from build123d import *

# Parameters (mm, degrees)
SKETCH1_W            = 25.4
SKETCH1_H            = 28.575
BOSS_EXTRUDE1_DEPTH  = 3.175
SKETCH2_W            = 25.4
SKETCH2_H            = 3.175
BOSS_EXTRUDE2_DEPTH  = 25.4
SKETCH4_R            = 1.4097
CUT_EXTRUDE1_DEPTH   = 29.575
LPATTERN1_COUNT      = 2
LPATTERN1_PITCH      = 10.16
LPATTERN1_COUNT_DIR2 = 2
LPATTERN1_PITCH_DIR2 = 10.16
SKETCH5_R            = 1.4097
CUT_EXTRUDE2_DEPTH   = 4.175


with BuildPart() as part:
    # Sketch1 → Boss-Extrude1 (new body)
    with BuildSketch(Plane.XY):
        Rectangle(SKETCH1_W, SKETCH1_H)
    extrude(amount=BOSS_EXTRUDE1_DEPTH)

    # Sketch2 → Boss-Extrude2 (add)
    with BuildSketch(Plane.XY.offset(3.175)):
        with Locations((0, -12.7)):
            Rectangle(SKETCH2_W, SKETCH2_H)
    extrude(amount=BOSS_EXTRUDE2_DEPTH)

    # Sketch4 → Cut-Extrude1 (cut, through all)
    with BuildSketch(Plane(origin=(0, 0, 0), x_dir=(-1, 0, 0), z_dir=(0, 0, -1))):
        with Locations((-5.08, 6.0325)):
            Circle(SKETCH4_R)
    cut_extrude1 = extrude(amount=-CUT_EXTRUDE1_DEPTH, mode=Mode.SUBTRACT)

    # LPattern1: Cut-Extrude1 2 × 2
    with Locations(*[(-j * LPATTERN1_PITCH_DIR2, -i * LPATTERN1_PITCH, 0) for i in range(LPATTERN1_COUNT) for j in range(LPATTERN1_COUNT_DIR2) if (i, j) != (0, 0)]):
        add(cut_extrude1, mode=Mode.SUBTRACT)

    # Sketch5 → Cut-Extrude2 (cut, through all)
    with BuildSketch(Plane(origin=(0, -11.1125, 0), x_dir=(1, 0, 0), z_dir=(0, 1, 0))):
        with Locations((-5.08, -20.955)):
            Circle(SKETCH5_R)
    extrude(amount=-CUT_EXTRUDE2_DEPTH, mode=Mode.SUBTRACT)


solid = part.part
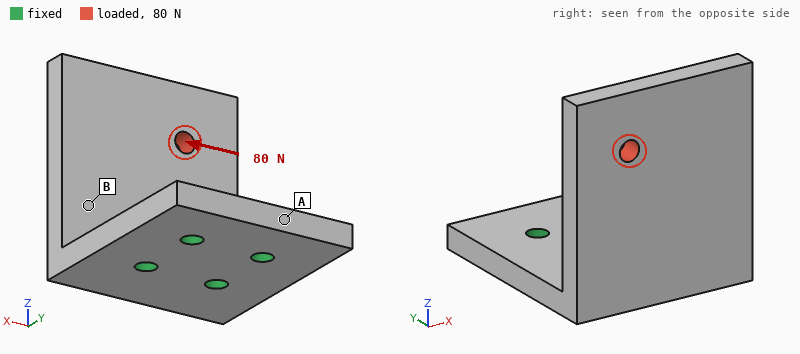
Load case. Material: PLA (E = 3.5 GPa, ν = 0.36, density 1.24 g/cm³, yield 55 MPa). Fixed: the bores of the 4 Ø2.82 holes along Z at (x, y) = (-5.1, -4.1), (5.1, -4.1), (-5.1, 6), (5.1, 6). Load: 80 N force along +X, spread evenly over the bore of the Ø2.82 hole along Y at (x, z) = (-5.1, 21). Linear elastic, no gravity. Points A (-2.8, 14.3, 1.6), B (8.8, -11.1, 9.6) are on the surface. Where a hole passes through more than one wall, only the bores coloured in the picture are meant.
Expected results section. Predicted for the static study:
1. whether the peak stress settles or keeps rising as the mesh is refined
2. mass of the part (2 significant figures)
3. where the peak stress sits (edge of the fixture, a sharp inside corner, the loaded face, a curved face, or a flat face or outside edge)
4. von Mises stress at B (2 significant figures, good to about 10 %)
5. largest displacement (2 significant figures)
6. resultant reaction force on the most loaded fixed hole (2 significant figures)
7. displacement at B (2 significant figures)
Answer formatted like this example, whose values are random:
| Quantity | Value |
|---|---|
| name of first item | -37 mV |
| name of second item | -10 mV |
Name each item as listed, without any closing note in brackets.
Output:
| Quantity | Value |
|---|---|
| whether the peak stress settles or keeps rising as the mesh is refined | keeps rising |
| mass of the part | 5.3 g |
| where the peak stress sits | edge of the fixture |
| von Mises stress at B | 6.7 MPa |
| largest displacement | 0.48 mm |
| resultant reaction force on the most loaded fixed hole | 130 N |
| displacement at B | 0.19 mm |
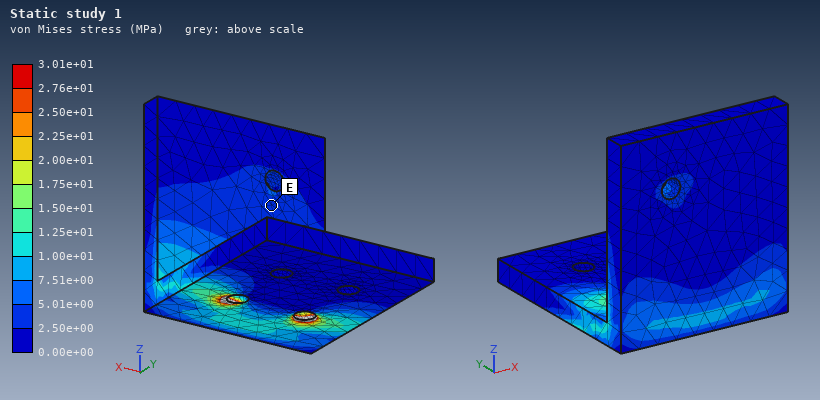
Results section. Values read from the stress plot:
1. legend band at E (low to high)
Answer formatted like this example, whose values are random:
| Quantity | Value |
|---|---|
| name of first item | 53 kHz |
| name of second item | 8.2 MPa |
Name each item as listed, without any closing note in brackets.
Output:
| Quantity | Value |
|---|---|
| legend band at E | 2.50e+00 to 5.01e+00 MPa |
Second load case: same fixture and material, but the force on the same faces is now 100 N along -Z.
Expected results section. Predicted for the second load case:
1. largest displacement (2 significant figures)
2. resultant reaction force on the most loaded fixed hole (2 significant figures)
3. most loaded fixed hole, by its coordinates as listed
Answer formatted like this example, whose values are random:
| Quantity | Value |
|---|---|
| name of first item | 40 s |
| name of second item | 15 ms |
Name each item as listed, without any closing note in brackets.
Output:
| Quantity | Value |
|---|---|
| largest displacement | 0.49 mm |
| resultant reaction force on the most loaded fixed hole | 98 N |
| most loaded fixed hole, by its coordinates as listed | (-5.1, -4.1) |
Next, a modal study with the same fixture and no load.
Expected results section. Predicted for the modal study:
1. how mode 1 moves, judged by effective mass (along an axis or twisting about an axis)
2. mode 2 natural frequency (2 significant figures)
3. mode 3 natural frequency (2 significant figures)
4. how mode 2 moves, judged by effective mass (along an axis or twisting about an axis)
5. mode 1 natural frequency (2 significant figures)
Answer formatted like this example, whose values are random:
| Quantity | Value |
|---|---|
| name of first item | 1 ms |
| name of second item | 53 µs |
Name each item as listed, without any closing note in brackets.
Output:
| Quantity | Value |
|---|---|
| how mode 1 moves, judged by effective mass | along Y |
| mode 2 natural frequency | 1700 Hz |
| mode 3 natural frequency | 2800 Hz |
| how mode 2 moves, judged by effective mass | along X |
| mode 1 natural frequency | 830 Hz |
